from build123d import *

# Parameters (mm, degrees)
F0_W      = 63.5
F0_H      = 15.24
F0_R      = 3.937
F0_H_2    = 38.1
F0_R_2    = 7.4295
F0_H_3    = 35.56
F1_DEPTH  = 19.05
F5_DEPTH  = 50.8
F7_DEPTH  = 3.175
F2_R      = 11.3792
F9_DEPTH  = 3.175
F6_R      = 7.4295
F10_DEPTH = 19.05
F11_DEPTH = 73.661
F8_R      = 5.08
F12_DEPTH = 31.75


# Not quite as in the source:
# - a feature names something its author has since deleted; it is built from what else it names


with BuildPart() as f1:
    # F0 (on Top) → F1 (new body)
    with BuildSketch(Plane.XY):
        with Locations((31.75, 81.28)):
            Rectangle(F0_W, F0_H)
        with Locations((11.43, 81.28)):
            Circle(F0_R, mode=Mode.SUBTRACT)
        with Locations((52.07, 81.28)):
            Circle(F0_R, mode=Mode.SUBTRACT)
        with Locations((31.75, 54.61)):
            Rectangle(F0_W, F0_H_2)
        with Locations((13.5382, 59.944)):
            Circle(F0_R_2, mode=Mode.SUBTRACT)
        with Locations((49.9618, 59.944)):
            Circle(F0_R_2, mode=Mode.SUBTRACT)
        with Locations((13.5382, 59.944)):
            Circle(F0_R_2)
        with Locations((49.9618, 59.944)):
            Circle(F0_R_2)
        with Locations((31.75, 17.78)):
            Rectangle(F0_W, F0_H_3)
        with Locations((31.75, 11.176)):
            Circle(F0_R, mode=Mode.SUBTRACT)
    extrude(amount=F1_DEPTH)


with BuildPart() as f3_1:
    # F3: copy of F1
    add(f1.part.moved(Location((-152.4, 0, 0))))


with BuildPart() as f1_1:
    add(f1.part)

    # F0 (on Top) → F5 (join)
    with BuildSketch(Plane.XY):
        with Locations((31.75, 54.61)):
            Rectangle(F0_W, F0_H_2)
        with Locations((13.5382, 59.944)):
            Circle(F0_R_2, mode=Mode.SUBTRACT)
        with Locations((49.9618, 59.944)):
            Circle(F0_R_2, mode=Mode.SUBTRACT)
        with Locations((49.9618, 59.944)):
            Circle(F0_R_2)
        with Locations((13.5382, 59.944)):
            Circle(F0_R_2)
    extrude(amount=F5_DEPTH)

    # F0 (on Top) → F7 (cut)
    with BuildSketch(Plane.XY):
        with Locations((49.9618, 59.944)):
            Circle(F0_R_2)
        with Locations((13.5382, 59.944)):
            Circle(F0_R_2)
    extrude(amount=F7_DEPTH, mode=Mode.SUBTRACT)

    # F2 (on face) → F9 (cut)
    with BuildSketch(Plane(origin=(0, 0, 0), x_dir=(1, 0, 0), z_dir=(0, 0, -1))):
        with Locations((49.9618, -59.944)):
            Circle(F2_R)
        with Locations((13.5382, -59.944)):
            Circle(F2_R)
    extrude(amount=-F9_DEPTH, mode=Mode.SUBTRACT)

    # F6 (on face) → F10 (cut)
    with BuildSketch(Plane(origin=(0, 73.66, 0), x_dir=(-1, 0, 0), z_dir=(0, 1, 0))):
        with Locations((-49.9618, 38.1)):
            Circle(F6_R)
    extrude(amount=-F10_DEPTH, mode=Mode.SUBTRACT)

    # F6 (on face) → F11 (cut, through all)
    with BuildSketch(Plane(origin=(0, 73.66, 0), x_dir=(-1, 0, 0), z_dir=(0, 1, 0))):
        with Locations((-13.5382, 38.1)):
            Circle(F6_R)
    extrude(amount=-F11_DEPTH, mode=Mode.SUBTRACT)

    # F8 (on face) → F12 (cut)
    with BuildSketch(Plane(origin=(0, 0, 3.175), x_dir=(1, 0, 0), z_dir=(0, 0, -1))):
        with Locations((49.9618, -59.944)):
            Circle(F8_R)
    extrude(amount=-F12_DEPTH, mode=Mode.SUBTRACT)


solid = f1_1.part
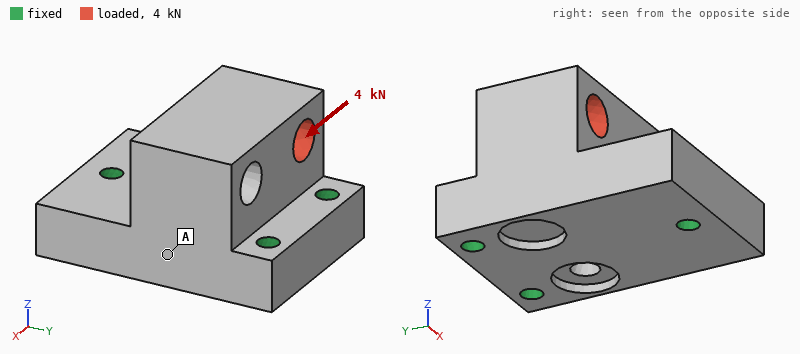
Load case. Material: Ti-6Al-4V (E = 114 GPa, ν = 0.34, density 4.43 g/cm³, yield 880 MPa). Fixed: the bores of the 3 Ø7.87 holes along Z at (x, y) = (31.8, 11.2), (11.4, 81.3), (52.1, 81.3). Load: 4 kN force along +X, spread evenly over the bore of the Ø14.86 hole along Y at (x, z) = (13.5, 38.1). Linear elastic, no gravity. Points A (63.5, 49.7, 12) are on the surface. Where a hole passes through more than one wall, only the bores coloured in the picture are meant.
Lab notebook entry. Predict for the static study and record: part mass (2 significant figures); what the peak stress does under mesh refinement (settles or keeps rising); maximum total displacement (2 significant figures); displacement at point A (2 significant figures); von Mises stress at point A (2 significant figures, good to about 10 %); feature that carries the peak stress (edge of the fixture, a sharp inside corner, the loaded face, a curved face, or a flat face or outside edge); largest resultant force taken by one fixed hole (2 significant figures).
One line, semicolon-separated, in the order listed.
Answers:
740 g; keeps rising; 8.4 µm; 3.8 µm; 2.6 MPa; edge of the fixture; 2.7 kN
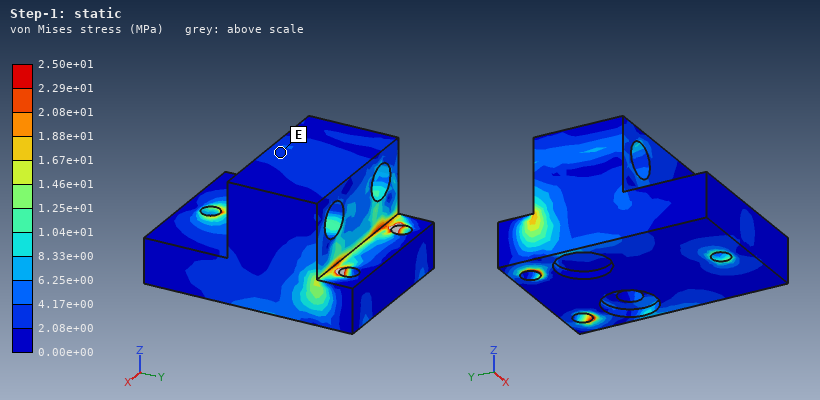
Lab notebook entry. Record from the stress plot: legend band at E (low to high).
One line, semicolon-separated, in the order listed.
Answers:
2.08e+00 to 4.17e+00 MPa
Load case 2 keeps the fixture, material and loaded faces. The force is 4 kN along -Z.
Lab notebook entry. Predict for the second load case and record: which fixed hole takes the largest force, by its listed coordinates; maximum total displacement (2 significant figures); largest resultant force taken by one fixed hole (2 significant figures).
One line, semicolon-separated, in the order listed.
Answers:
(11.4, 81.3); 6.8 µm; 2.6 kN
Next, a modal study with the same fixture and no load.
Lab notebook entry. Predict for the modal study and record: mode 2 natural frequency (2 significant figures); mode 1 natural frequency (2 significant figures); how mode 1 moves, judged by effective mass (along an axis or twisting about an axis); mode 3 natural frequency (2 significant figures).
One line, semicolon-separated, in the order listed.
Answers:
7800 Hz; 7200 Hz; along X; 13 kHz
